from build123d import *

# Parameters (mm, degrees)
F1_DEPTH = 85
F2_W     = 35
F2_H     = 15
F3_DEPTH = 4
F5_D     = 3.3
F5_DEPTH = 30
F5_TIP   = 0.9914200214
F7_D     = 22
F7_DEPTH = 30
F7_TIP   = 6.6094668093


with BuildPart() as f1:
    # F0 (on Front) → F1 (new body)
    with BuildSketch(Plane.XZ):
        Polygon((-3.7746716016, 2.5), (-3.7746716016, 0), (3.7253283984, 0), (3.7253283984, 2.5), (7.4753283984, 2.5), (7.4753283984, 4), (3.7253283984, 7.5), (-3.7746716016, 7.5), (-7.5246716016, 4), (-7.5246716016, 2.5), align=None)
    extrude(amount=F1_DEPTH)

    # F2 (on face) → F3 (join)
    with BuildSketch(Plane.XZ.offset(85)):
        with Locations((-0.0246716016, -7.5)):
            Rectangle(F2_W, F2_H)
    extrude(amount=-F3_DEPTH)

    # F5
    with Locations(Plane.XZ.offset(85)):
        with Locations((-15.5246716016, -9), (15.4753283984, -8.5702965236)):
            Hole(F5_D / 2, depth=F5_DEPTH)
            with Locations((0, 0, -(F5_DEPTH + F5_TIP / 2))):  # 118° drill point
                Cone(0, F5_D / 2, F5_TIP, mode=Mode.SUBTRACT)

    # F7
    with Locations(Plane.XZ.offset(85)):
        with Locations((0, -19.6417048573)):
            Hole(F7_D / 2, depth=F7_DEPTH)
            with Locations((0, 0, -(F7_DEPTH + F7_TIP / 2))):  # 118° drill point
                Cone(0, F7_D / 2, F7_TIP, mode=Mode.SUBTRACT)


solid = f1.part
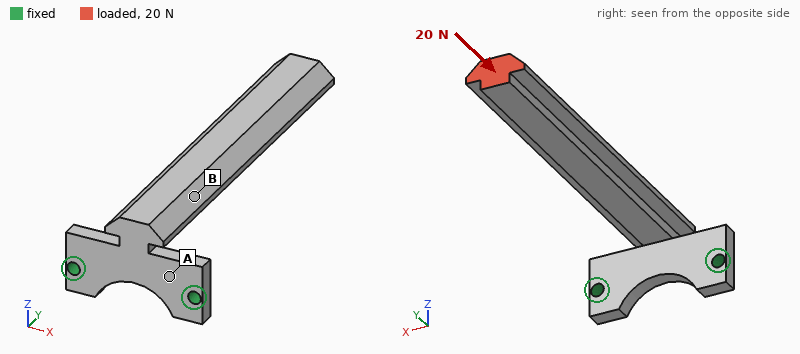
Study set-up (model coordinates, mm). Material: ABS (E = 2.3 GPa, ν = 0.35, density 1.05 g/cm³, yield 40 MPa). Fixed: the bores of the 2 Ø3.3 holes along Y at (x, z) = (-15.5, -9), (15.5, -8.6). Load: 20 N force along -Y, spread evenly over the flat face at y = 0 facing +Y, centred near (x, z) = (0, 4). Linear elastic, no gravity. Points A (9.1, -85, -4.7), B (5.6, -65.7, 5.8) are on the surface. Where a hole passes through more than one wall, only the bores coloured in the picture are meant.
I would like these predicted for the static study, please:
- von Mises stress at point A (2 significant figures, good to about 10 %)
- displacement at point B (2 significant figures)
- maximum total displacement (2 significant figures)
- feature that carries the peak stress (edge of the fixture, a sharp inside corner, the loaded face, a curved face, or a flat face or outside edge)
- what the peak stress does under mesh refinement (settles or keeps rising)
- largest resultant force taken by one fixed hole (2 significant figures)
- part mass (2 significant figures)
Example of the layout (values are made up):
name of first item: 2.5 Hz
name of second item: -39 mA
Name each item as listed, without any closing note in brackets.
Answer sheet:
von Mises stress at point A: 3.2 MPa
displacement at point B: 0.28 mm
maximum total displacement: 1.1 mm
feature that carries the peak stress: edge of the fixture
what the peak stress does under mesh refinement: keeps rising
largest resultant force taken by one fixed hole: 10 N
part mass: 8.9 g
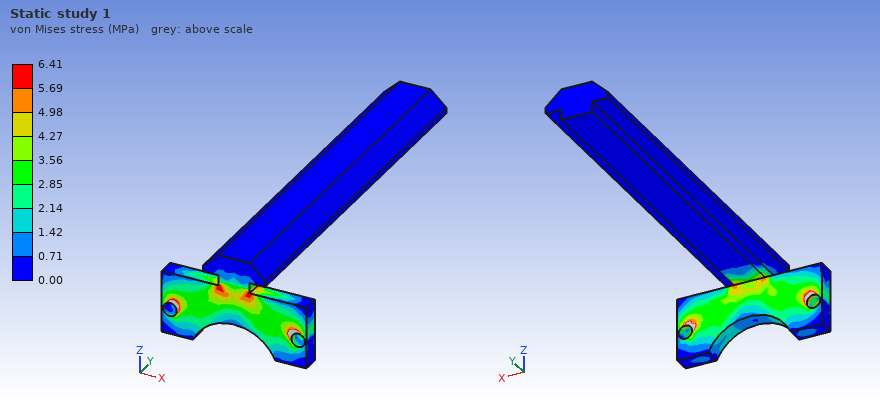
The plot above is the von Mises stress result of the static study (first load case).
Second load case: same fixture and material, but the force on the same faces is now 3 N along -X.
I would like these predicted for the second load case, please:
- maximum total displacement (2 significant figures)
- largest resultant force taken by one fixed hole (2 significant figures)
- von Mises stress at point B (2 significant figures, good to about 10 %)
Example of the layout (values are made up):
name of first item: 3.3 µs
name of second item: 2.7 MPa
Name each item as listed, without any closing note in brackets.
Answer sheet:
maximum total displacement: 1.0 mm
largest resultant force taken by one fixed hole: 11 N
von Mises stress at point B: 1.1 MPa
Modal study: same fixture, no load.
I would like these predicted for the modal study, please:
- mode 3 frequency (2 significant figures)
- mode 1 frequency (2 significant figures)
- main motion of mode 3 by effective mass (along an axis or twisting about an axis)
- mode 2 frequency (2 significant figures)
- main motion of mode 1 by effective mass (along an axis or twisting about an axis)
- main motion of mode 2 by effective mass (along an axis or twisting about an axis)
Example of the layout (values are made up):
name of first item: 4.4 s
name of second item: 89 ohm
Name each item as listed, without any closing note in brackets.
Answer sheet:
mode 3 frequency: 880 Hz
mode 1 frequency: 120 Hz
main motion of mode 3 by effective mass: along Y
mode 2 frequency: 180 Hz
main motion of mode 1 by effective mass: along Z
main motion of mode 2 by effective mass: along X
